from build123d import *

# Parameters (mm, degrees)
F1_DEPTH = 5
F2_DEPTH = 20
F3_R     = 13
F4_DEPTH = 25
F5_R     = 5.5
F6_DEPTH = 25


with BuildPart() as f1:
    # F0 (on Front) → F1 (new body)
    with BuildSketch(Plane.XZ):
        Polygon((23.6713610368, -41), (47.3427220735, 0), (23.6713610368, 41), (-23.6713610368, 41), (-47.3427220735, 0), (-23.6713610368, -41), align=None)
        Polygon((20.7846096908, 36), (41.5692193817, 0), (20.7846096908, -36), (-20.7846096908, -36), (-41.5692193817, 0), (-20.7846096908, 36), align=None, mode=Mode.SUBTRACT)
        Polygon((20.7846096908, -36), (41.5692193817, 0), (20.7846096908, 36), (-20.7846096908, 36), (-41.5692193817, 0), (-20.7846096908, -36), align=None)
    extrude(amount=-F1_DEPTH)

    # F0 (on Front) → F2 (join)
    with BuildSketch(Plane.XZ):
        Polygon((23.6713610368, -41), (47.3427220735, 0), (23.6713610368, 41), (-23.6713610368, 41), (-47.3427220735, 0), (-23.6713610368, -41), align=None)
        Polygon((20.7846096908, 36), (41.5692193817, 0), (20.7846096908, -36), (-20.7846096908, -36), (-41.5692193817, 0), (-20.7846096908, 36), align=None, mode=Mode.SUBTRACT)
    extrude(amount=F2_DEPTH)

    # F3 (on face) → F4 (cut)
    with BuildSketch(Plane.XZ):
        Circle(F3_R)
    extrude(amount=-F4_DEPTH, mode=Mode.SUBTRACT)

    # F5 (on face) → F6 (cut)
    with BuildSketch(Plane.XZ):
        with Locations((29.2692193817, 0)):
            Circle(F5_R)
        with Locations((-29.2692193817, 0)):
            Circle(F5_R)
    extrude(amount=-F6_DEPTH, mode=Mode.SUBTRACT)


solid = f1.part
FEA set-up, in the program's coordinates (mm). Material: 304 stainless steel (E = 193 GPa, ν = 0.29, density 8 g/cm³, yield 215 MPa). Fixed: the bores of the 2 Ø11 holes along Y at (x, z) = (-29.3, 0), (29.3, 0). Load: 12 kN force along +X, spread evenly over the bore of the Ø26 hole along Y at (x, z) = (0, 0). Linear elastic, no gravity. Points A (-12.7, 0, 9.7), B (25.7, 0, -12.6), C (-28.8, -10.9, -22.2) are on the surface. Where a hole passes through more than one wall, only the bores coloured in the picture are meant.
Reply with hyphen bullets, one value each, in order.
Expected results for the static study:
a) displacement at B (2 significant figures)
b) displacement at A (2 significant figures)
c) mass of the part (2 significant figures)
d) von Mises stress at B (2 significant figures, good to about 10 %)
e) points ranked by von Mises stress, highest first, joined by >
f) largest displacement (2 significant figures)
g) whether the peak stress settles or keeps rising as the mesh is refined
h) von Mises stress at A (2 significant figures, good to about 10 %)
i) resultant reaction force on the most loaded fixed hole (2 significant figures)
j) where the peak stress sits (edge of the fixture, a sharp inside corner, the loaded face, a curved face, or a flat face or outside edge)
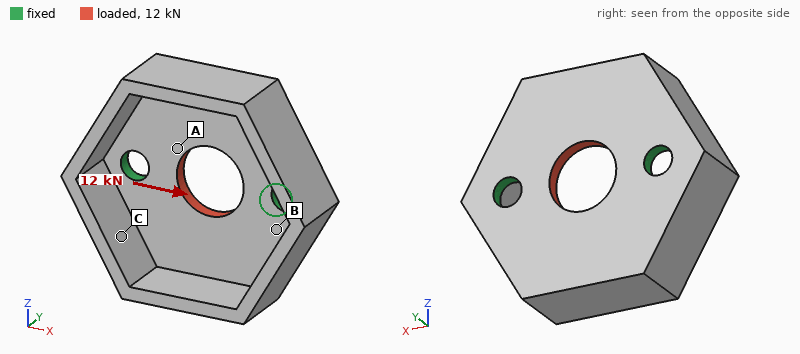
- 2.3 µm
- 3.9 µm
- 420 g
- 21 MPa
- A > B > C
- 5.8 µm
- keeps rising
- 41 MPa
- 6.0 kN
- edge of the fixture
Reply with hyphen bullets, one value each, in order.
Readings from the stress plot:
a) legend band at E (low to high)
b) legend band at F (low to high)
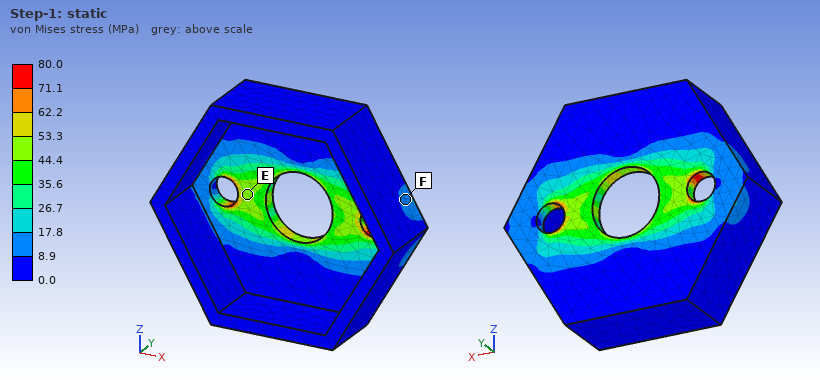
- 44.4 to 53.3 MPa
- 8.9 to 17.8 MPa
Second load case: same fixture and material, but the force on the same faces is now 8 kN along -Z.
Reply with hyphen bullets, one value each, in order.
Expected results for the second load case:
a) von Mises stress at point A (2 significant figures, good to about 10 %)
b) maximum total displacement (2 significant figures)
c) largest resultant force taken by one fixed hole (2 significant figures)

- 25 MPa
- 4.7 µm
- 4.0 kN
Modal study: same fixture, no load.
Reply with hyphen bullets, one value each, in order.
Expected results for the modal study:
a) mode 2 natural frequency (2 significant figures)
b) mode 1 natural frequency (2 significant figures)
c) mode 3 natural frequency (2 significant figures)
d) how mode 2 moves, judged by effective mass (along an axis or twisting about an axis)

- 3300 Hz
- 2300 Hz
- 4000 Hz
- along Y
